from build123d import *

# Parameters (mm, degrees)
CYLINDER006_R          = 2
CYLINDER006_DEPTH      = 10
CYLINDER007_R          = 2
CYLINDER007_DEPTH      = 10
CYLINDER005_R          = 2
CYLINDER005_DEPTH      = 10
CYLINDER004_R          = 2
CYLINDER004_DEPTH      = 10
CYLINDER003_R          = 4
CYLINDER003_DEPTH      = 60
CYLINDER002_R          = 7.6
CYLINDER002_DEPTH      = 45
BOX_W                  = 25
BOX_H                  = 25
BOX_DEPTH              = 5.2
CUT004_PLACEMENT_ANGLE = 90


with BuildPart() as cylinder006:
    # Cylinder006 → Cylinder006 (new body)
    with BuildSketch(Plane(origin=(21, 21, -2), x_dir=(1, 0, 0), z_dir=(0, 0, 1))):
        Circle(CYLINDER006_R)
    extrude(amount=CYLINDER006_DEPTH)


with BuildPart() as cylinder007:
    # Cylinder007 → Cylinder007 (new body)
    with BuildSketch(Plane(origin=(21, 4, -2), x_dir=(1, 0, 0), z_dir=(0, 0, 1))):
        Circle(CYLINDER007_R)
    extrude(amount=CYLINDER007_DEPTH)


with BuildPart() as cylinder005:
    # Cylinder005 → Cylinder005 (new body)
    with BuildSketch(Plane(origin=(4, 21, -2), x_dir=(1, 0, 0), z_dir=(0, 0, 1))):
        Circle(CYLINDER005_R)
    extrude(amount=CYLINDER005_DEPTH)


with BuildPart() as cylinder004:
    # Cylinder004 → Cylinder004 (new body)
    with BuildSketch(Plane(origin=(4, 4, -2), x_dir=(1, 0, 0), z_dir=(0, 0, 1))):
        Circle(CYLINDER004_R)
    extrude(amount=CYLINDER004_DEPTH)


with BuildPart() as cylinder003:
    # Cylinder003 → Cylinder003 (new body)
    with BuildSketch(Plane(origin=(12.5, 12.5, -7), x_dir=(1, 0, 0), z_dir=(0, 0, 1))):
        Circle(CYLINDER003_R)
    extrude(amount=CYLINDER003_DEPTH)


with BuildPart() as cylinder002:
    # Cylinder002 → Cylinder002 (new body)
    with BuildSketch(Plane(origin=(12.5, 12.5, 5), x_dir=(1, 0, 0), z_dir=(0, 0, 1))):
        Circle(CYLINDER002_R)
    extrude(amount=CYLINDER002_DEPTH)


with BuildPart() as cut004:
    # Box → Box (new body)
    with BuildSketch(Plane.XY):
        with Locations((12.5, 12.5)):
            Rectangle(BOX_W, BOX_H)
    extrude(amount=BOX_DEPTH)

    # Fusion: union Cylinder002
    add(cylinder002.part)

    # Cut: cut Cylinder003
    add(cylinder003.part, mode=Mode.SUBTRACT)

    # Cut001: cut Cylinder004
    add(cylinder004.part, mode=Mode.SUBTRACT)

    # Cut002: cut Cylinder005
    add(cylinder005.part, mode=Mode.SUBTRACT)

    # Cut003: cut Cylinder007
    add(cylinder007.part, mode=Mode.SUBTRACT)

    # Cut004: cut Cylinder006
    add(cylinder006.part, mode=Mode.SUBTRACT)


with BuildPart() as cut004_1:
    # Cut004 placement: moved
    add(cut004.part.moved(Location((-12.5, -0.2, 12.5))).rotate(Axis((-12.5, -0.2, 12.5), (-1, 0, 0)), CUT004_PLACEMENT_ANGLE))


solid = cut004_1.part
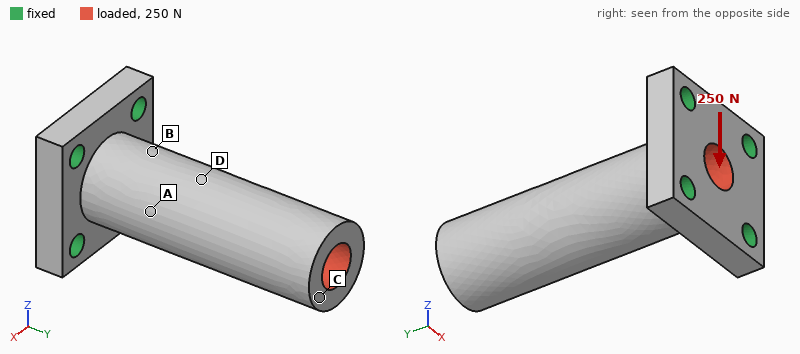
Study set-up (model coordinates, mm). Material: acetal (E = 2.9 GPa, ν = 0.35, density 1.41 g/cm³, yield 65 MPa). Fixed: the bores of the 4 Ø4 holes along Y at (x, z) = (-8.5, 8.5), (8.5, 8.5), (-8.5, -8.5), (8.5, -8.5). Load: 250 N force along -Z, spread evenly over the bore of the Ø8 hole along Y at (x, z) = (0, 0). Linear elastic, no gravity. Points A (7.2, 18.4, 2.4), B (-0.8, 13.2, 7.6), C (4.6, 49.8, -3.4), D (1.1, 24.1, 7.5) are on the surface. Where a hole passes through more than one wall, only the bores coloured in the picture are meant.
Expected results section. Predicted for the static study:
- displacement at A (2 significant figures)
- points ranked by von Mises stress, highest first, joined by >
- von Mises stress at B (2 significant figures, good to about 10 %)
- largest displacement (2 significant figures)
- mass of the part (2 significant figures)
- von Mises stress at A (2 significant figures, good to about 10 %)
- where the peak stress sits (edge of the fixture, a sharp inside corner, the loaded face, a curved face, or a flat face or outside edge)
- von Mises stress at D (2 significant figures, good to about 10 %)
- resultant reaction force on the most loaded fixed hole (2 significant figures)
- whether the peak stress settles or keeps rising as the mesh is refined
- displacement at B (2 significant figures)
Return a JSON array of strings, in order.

["0.15 mm", "B > D > A > C", "10 MPa", "0.64 mm", "12 g", "3.9 MPa", "edge of the fixture", "5.1 MPa", "200 N", "keeps rising", "0.11 mm"]
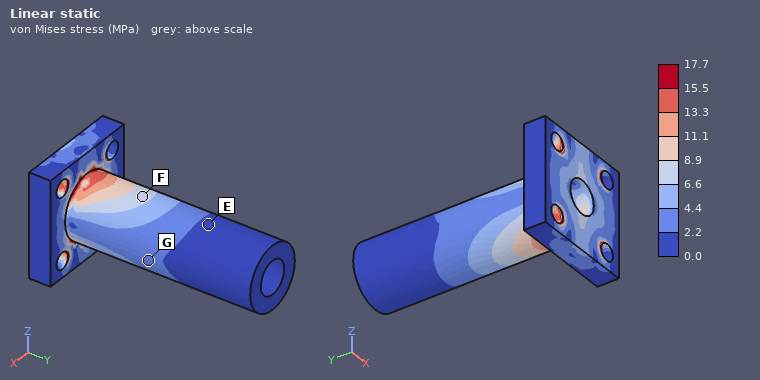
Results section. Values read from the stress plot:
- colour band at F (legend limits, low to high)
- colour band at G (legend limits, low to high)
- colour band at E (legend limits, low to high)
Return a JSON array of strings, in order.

["6.6 to 8.9 MPa", "2.2 to 4.4 MPa", "0.0 to 2.2 MPa"]
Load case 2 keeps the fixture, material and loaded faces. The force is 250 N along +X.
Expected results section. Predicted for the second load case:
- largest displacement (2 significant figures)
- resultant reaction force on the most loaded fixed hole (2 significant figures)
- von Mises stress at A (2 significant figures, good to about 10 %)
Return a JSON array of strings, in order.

["0.64 mm", "200 N", "7.3 MPa"]
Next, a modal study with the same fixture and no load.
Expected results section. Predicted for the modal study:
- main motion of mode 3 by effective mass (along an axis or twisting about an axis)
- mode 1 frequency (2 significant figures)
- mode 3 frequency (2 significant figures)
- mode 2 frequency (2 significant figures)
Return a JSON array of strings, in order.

["twisting about Y", "1300 Hz", "4700 Hz", "1300 Hz"]
